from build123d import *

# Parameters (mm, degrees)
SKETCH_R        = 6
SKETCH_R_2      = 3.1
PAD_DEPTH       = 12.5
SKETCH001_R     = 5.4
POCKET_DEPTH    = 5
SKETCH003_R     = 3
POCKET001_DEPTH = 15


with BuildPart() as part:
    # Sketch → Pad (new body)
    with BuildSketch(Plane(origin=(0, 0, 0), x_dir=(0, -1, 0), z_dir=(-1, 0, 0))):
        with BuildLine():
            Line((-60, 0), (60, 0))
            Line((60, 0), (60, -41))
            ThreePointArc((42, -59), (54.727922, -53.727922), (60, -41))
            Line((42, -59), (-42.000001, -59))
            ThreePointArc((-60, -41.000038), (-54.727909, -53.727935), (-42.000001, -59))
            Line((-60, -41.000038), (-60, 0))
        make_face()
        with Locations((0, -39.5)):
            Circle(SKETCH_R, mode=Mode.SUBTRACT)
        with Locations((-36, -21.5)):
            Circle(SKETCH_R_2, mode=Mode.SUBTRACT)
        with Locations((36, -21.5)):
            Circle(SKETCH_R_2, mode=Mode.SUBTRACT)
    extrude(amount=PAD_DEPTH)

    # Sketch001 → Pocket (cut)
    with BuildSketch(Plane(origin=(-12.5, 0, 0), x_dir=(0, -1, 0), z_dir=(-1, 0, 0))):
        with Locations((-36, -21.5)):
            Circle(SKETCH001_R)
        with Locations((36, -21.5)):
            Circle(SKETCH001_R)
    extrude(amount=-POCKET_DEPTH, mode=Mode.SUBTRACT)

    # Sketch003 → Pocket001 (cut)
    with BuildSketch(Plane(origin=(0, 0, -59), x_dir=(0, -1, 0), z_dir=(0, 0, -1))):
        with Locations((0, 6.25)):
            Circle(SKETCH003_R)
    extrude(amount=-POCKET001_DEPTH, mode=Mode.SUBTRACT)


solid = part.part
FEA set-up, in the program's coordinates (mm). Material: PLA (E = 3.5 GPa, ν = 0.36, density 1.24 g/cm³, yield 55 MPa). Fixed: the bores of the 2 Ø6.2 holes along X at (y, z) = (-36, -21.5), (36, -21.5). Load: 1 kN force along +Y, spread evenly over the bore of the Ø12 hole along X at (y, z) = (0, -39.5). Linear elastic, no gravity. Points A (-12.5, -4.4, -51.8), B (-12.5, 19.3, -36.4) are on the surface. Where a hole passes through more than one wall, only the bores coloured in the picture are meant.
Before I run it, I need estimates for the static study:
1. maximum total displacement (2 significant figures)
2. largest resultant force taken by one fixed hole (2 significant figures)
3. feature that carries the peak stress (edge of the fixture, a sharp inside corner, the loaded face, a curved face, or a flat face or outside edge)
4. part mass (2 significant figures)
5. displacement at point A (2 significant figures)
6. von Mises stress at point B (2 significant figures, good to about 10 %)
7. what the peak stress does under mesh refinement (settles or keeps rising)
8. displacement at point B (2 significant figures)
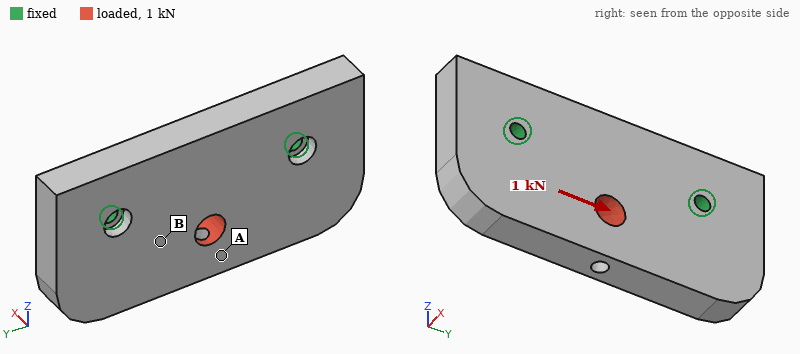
32 µm
550 N
edge of the fixture
100 g
23 µm
1.5 MPa
keeps rising
18 µm
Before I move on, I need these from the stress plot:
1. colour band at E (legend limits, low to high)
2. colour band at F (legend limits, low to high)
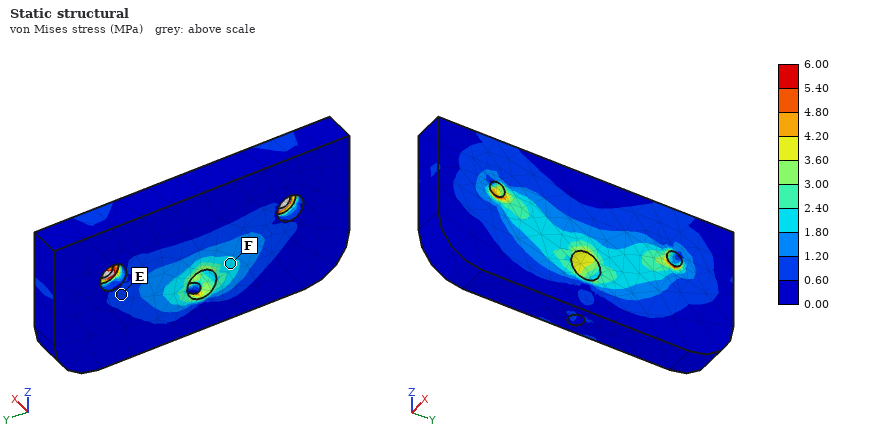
0.60 to 1.20 MPa
1.80 to 2.40 MPa
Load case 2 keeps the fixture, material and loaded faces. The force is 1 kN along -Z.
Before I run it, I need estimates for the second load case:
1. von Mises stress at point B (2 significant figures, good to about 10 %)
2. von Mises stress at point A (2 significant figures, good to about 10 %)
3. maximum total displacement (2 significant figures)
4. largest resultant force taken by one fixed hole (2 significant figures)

1.4 MPa
3.2 MPa
72 µm
510 N
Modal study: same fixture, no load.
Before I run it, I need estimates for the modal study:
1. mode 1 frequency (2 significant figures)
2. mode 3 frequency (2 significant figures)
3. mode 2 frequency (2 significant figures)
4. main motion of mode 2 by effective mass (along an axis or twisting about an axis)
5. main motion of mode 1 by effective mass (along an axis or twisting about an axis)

1100 Hz
2100 Hz
1900 Hz
twisting about Z
along X
